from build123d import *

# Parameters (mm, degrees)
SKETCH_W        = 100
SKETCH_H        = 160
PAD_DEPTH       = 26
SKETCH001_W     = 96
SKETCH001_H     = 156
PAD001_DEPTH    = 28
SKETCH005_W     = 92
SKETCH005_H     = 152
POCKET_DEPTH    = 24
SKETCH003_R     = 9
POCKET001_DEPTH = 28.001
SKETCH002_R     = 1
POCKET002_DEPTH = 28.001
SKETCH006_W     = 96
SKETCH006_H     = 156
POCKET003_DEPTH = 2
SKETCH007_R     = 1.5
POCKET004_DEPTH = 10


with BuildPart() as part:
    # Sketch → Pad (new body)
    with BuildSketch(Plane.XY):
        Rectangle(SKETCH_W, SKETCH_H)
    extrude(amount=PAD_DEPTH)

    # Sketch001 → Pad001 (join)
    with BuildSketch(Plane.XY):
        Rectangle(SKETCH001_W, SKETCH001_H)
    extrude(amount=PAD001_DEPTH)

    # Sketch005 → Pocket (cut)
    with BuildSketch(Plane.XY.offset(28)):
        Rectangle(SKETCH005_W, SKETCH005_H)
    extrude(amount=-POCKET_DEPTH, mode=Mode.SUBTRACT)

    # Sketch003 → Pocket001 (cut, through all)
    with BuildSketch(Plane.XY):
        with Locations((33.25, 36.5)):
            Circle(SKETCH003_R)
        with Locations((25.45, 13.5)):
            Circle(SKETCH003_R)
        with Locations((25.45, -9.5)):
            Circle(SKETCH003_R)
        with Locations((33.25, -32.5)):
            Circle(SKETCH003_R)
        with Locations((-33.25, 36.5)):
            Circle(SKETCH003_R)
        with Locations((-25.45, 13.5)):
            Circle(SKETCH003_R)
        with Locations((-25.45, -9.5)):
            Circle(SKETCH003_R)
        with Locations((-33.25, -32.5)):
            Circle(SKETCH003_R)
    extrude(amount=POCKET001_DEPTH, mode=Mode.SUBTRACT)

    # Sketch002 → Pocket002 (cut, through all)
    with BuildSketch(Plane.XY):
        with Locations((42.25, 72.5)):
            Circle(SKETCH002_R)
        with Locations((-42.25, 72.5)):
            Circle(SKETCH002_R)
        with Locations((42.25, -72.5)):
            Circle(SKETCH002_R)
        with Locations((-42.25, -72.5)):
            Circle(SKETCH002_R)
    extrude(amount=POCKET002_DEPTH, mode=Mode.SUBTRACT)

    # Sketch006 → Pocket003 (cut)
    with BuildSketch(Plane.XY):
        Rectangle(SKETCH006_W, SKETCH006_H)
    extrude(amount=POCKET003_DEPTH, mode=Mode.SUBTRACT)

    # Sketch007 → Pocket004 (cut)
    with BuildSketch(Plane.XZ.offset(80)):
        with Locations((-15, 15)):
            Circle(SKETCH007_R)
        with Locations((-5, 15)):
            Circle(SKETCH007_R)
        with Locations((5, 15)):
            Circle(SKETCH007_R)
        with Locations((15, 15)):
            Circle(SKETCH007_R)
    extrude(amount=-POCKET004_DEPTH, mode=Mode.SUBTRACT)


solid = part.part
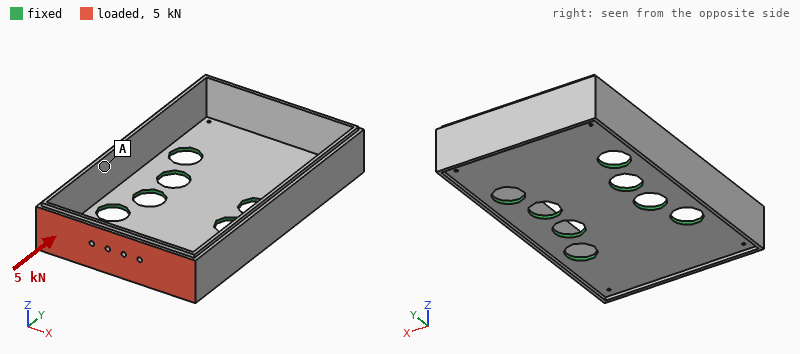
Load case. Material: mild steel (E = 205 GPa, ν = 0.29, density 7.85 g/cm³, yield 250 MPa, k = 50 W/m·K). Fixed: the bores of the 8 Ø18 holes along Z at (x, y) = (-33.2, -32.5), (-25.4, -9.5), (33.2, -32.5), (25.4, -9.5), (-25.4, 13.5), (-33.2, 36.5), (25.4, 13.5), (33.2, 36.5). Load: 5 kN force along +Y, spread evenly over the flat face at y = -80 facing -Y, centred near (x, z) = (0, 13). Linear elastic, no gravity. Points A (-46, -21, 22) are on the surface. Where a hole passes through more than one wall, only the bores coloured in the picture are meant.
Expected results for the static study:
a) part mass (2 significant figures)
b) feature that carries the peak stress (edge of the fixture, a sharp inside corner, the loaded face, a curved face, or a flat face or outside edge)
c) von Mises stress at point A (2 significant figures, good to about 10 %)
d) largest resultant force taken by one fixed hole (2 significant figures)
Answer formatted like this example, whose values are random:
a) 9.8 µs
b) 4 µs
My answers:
a) 600 g
b) a flat face or outside edge
c) 17 MPa
d) 1.5 kN
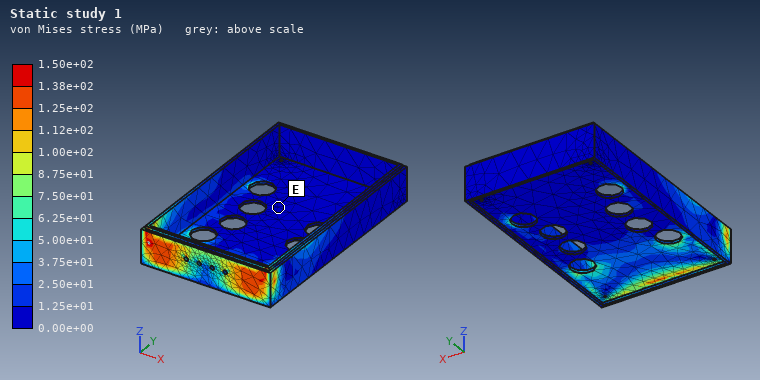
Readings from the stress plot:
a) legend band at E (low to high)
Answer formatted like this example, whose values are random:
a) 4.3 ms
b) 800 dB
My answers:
a) 0.00e+00 to 1.25e+01 MPa
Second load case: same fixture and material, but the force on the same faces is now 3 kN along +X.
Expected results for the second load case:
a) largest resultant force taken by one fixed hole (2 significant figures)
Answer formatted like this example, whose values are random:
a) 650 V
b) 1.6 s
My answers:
a) 2.4 kN
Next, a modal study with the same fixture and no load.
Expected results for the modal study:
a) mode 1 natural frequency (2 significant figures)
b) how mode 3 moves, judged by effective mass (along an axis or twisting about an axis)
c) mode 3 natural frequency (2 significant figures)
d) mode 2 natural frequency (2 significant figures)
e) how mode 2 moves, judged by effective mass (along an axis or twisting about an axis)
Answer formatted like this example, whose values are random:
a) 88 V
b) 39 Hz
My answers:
a) 2100 Hz
b) along Z
c) 2400 Hz
d) 2300 Hz
e) along X
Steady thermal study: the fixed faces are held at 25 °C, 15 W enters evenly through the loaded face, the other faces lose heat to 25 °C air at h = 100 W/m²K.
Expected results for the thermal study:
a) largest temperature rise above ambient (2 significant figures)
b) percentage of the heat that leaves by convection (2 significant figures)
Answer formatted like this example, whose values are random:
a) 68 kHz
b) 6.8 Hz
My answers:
a) 17 K
b) 83 %
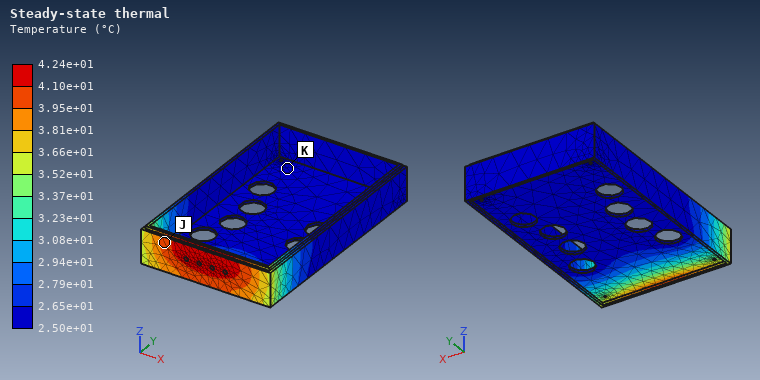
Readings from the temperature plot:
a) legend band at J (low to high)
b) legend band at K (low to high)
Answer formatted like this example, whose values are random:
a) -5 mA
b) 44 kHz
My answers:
a) 3.95e+01 to 4.10e+01 °C
b) 2.50e+01 to 2.65e+01 °C
